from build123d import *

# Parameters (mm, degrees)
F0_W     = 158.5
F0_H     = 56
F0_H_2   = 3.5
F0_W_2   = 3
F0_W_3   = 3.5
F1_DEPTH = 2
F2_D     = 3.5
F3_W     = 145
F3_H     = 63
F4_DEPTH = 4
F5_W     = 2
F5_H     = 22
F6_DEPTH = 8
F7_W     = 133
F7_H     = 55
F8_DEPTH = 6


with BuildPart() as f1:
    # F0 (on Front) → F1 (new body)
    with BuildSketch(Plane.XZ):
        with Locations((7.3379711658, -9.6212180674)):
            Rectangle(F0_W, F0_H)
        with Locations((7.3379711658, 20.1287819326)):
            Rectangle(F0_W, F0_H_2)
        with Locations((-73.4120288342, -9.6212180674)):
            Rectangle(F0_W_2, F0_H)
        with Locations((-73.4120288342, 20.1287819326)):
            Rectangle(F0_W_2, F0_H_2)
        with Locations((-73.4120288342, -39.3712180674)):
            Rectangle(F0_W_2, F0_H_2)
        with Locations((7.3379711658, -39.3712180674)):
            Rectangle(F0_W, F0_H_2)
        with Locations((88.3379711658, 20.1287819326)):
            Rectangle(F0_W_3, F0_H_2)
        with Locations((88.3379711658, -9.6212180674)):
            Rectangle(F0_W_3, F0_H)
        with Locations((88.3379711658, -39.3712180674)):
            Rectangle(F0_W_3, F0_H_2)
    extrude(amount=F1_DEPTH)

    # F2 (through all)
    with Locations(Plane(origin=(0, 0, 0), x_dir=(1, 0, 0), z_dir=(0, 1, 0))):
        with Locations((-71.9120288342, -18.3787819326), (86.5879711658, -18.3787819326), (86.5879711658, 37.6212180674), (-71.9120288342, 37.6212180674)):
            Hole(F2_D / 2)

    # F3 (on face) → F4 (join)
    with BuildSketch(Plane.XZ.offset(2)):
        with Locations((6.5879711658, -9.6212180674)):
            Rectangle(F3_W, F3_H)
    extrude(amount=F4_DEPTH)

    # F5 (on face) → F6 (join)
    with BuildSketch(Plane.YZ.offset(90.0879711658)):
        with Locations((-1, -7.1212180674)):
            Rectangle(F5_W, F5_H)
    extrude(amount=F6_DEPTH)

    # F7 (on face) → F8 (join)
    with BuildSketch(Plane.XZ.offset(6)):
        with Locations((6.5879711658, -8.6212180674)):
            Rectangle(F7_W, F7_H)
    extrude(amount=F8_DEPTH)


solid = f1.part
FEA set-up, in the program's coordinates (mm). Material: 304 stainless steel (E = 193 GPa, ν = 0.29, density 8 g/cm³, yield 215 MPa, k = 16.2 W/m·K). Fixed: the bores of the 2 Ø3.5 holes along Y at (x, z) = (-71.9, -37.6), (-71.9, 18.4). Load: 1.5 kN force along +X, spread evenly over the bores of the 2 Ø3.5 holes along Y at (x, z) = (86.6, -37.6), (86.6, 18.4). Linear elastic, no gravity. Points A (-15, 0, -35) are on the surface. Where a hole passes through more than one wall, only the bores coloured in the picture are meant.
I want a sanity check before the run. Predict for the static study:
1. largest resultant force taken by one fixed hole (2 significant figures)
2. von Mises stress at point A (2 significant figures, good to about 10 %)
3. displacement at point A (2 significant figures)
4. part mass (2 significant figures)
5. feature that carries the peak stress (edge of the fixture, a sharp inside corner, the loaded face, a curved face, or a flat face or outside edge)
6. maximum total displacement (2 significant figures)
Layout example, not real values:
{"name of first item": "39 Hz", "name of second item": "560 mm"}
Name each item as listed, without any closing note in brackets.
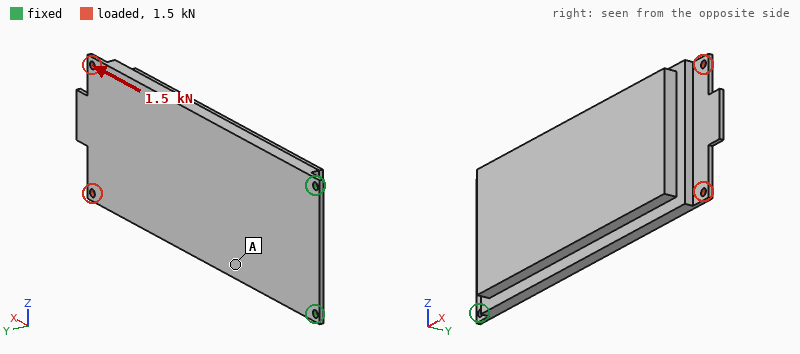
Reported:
{"largest resultant force taken by one fixed hole": "780 N", "von Mises stress at point A": "7.1 MPa", "displacement at point A": "13 µm", "part mass": "810 g", "feature that carries the peak stress": "the loaded face", "maximum total displacement": "83 µm"}
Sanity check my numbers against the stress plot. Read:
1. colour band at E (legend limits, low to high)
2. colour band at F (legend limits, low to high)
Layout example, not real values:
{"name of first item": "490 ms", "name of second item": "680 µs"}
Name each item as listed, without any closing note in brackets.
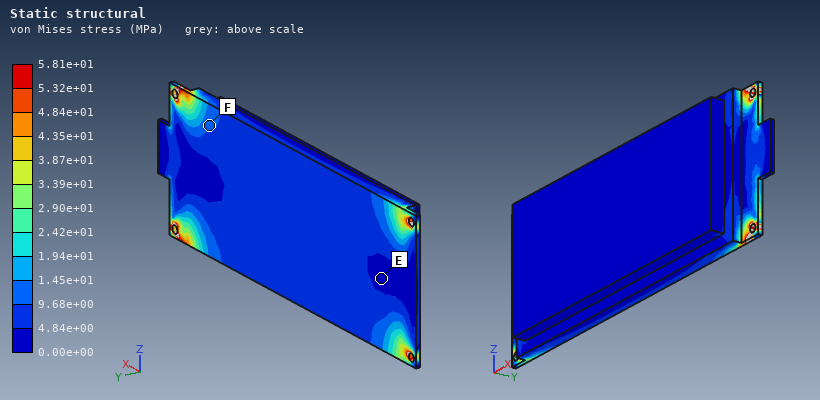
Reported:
{"colour band at E": "0.00e+00 to 4.84e+00 MPa", "colour band at F": "9.68e+00 to 1.45e+01 MPa"}
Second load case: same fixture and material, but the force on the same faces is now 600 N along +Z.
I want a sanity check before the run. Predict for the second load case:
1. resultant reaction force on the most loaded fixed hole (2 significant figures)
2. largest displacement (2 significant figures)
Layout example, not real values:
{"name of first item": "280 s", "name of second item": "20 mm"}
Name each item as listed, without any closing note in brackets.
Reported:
{"resultant reaction force on the most loaded fixed hole": "1.7 kN", "largest displacement": "65 µm"}
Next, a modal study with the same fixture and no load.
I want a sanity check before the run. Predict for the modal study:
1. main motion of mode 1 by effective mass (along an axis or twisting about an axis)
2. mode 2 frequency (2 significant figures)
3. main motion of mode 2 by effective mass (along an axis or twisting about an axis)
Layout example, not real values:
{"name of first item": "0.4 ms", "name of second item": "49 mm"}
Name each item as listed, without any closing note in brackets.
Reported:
{"main motion of mode 1 by effective mass": "along Y", "mode 2 frequency": "1100 Hz", "main motion of mode 2 by effective mass": "along Z"}
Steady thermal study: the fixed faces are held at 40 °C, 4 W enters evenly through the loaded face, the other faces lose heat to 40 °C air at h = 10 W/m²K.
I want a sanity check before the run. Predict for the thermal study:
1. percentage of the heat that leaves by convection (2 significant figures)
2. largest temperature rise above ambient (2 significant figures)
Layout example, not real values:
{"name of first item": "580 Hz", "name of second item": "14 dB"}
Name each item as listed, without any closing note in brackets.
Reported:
{"percentage of the heat that leaves by convection": "88 %", "largest temperature rise above ambient": "84 K"}
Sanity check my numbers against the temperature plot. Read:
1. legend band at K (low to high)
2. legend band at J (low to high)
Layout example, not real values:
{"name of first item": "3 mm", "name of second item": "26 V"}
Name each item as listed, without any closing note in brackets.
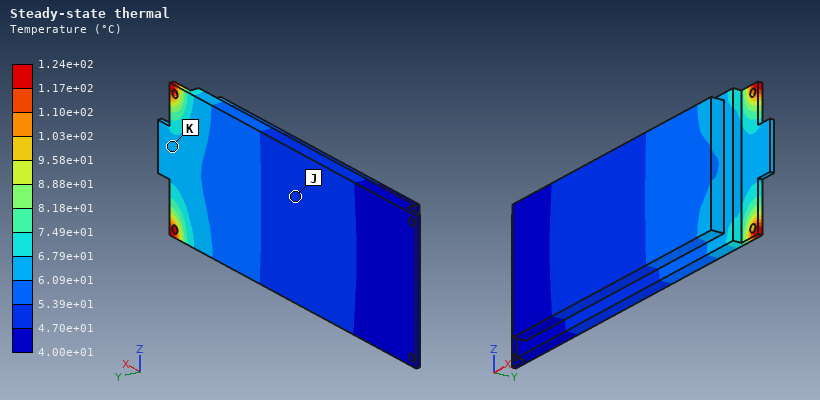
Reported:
{"legend band at K": "6.09e+01 to 6.79e+01 °C", "legend band at J": "4.70e+01 to 5.39e+01 °C"}
